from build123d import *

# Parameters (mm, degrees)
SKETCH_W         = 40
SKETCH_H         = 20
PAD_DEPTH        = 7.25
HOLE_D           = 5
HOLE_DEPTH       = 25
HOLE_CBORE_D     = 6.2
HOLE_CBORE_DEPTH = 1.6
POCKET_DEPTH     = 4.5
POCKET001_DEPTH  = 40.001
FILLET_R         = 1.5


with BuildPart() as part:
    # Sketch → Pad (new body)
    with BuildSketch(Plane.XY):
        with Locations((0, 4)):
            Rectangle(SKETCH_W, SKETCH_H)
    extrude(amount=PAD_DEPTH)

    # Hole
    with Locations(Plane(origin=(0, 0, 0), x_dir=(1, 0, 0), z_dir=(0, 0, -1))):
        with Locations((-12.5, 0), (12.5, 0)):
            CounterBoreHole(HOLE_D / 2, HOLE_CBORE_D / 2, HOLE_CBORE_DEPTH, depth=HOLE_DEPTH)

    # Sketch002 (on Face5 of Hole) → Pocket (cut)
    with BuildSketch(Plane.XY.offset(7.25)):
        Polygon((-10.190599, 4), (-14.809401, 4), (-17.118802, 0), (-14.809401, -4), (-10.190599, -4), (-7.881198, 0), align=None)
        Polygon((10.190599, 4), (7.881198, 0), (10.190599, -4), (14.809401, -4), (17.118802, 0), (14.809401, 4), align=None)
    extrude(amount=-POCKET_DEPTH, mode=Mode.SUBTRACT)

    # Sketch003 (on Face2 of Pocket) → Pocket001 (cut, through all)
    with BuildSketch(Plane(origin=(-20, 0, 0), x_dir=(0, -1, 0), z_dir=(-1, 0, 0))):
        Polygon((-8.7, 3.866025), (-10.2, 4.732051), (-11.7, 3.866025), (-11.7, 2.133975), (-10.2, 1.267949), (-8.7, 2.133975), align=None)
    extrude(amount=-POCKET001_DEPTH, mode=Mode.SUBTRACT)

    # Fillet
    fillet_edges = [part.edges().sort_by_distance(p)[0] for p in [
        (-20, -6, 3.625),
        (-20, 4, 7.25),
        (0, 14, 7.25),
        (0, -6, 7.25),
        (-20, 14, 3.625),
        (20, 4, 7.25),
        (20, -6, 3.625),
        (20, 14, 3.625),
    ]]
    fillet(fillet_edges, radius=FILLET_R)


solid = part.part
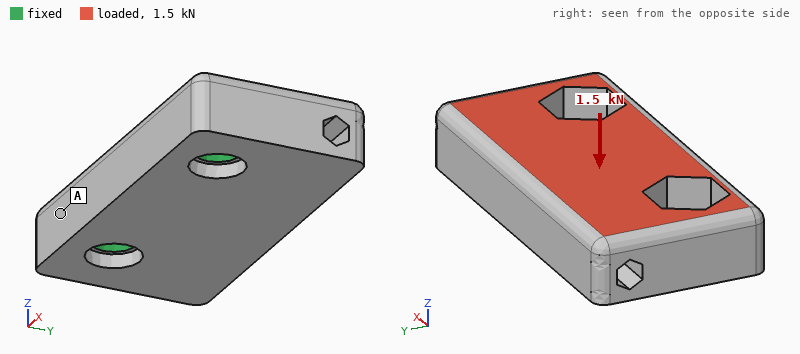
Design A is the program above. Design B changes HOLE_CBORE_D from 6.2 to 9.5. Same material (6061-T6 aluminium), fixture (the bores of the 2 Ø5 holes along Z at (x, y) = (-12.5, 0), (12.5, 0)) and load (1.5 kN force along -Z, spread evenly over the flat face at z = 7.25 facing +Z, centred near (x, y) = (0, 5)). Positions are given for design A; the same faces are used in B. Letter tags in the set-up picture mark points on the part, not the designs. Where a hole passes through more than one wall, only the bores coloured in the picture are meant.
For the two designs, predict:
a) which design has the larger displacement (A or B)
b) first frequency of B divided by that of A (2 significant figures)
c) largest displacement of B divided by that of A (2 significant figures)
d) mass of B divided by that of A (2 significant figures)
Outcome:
B
0.87
1.3
0.97
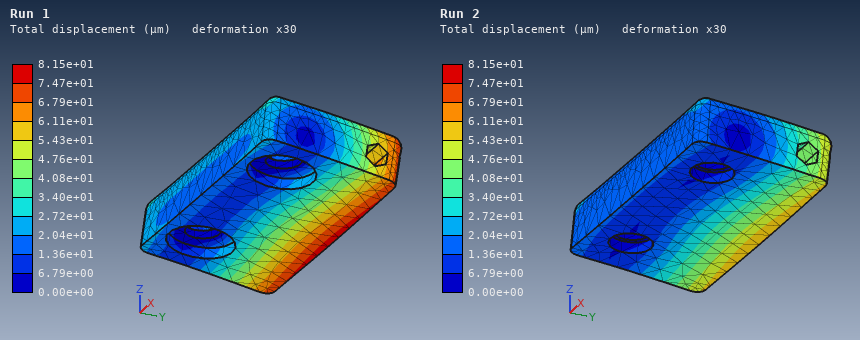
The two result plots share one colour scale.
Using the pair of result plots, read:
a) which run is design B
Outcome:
Run 1
